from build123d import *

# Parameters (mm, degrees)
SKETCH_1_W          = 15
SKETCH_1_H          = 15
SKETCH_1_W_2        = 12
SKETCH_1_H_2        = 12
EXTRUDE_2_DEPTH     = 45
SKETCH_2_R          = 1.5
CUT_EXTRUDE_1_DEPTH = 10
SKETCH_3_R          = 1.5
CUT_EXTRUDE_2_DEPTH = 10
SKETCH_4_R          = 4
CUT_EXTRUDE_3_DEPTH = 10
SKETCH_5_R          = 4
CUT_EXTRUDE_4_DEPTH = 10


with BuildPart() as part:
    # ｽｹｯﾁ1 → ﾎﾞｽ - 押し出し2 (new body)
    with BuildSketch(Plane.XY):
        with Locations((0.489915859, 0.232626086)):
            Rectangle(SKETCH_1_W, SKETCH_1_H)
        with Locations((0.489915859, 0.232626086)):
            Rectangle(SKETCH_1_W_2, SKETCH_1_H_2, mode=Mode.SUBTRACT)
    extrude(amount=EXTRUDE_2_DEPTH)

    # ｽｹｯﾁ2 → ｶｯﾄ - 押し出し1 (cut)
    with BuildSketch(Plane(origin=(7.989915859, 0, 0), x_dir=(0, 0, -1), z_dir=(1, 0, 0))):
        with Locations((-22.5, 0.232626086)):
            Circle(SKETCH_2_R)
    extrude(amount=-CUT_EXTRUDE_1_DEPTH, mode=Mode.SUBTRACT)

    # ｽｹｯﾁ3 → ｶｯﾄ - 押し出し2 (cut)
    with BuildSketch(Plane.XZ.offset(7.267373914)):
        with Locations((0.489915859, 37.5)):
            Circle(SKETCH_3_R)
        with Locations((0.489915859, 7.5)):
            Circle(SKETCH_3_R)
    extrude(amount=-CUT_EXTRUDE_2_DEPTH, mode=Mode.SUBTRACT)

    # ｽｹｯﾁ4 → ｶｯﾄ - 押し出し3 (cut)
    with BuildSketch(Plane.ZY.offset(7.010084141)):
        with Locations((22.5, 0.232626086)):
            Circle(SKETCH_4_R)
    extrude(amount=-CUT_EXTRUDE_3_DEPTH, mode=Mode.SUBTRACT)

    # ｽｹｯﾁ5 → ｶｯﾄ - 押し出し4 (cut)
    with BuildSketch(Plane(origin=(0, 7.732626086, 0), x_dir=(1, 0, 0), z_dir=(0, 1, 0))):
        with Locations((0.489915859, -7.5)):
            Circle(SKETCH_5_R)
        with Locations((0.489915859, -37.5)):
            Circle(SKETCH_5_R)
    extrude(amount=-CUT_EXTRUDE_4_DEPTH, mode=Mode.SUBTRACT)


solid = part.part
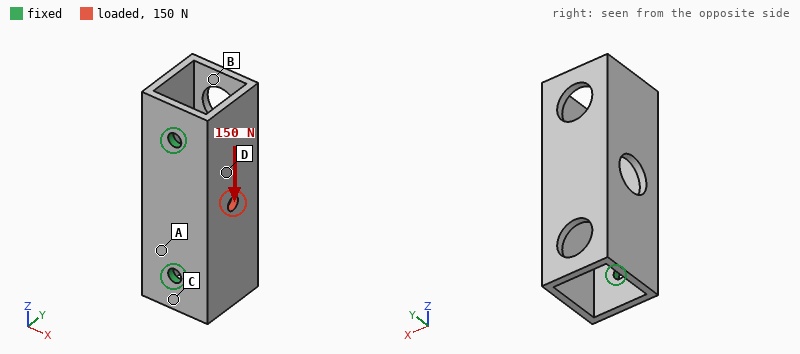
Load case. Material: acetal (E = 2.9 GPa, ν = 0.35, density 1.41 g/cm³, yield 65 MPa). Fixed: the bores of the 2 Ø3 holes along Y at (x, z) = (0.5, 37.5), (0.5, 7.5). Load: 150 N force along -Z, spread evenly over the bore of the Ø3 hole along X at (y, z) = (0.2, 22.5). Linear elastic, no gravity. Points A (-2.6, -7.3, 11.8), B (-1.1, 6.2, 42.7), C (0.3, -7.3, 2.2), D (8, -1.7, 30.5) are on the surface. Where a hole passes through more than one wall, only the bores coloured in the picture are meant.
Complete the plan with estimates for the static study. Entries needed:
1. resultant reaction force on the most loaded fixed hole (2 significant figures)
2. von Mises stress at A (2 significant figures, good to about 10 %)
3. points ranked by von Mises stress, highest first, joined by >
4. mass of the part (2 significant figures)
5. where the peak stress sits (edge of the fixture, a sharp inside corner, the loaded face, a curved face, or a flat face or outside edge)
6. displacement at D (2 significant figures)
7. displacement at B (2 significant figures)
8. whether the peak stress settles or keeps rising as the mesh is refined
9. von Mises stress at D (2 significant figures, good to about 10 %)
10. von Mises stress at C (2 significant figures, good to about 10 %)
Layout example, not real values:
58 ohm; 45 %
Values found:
87 N; 3.3 MPa; C > D > A > B; 4.8 g; edge of the fixture; 0.060 mm; 0.12 mm; keeps rising; 6.1 MPa; 8.9 MPa
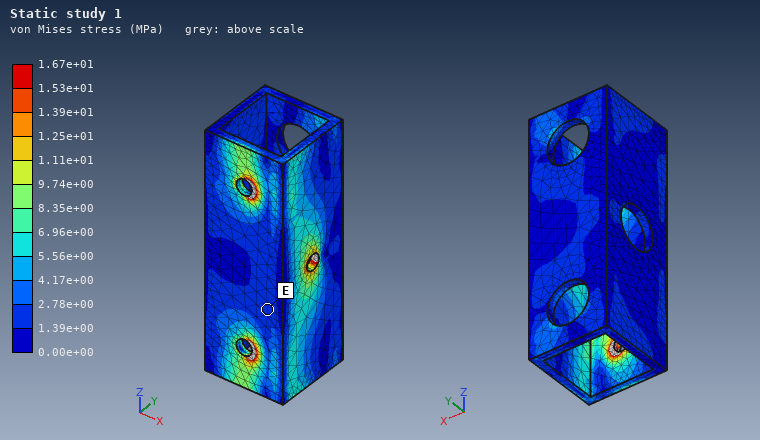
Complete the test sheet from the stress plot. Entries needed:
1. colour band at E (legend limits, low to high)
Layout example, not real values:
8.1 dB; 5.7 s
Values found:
1.39e+00 to 2.78e+00 MPa
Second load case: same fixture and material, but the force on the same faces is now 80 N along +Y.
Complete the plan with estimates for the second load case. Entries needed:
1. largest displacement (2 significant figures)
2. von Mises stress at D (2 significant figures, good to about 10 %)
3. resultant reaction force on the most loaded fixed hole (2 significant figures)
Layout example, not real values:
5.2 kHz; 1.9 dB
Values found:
0.50 mm; 4.1 MPa; 43 N
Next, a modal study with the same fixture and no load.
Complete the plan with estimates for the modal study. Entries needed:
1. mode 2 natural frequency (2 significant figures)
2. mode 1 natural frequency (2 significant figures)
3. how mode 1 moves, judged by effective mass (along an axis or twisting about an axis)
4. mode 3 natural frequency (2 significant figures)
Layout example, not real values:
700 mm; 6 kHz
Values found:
2500 Hz; 840 Hz; along X; 2500 Hz
